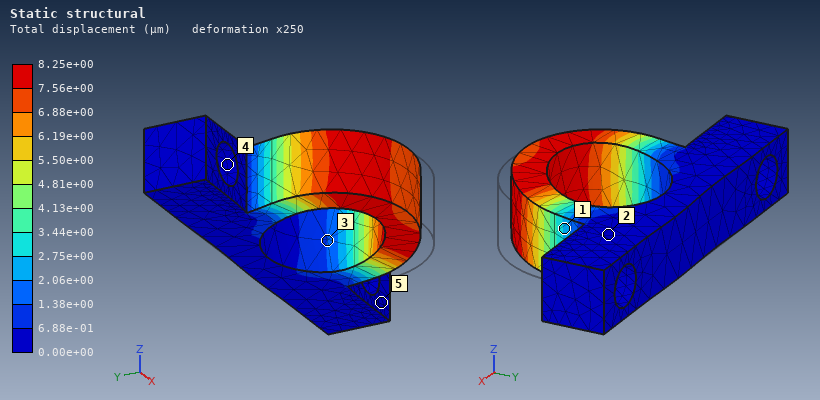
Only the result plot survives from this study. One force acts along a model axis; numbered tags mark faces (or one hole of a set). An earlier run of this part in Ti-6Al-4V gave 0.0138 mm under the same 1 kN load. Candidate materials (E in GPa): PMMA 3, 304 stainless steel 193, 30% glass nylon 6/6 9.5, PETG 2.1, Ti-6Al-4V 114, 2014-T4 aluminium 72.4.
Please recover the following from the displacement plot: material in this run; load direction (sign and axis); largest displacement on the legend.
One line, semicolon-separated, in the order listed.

304 stainless steel; -X; 8.25e+00 µm
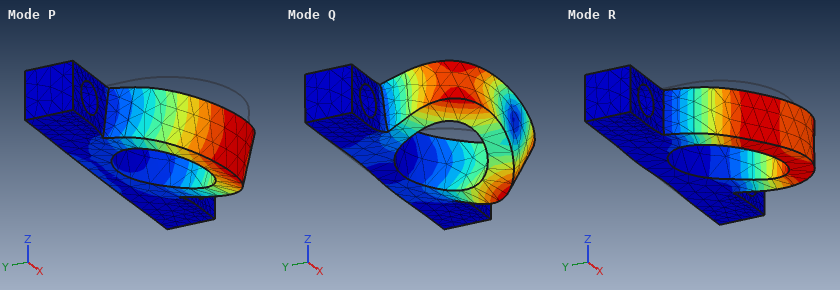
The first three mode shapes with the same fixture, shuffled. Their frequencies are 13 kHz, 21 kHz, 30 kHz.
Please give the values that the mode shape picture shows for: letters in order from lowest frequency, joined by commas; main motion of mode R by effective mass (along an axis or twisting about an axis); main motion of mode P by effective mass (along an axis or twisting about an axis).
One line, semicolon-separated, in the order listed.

P, R, Q; along X; along Z
